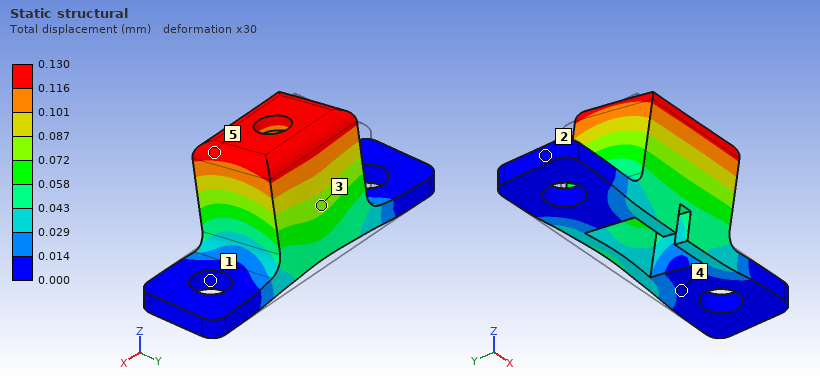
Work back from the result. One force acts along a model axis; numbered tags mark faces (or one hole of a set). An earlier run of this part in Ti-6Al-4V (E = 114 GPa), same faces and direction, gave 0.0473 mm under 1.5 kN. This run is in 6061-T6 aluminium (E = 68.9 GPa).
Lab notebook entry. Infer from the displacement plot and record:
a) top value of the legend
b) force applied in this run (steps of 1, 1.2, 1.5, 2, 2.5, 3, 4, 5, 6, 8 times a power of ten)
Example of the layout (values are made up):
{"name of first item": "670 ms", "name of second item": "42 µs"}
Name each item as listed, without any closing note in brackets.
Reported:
{"top value of the legend": "0.130 mm", "force applied in this run": "2.5 kN"}
